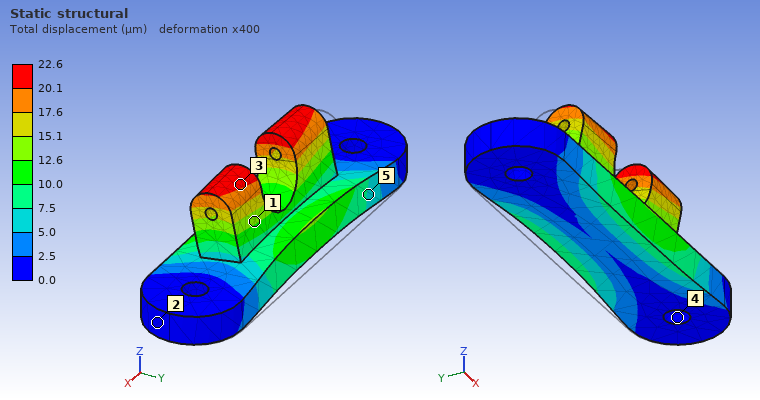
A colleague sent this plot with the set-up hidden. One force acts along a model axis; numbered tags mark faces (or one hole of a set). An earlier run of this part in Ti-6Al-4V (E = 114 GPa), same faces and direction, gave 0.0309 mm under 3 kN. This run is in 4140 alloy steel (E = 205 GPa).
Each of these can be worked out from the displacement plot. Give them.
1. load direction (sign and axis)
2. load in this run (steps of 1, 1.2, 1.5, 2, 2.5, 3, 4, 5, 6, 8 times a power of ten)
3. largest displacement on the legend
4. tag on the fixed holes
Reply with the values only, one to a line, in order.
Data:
-Y
4 kN
22.6 µm
4
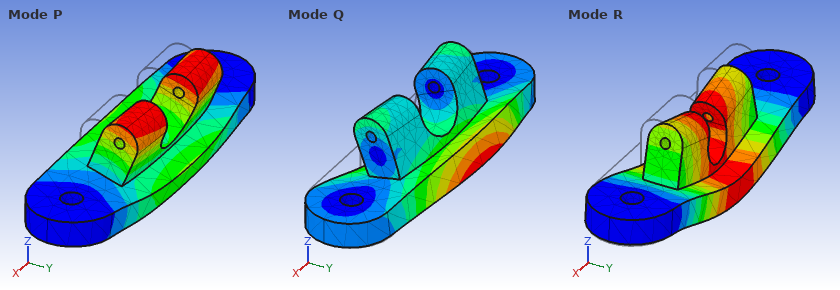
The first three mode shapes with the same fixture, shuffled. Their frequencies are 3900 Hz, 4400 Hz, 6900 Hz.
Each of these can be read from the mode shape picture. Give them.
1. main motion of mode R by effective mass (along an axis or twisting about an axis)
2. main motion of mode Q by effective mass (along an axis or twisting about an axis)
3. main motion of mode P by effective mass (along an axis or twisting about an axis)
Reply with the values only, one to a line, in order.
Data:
along Z
along Y
along Y
